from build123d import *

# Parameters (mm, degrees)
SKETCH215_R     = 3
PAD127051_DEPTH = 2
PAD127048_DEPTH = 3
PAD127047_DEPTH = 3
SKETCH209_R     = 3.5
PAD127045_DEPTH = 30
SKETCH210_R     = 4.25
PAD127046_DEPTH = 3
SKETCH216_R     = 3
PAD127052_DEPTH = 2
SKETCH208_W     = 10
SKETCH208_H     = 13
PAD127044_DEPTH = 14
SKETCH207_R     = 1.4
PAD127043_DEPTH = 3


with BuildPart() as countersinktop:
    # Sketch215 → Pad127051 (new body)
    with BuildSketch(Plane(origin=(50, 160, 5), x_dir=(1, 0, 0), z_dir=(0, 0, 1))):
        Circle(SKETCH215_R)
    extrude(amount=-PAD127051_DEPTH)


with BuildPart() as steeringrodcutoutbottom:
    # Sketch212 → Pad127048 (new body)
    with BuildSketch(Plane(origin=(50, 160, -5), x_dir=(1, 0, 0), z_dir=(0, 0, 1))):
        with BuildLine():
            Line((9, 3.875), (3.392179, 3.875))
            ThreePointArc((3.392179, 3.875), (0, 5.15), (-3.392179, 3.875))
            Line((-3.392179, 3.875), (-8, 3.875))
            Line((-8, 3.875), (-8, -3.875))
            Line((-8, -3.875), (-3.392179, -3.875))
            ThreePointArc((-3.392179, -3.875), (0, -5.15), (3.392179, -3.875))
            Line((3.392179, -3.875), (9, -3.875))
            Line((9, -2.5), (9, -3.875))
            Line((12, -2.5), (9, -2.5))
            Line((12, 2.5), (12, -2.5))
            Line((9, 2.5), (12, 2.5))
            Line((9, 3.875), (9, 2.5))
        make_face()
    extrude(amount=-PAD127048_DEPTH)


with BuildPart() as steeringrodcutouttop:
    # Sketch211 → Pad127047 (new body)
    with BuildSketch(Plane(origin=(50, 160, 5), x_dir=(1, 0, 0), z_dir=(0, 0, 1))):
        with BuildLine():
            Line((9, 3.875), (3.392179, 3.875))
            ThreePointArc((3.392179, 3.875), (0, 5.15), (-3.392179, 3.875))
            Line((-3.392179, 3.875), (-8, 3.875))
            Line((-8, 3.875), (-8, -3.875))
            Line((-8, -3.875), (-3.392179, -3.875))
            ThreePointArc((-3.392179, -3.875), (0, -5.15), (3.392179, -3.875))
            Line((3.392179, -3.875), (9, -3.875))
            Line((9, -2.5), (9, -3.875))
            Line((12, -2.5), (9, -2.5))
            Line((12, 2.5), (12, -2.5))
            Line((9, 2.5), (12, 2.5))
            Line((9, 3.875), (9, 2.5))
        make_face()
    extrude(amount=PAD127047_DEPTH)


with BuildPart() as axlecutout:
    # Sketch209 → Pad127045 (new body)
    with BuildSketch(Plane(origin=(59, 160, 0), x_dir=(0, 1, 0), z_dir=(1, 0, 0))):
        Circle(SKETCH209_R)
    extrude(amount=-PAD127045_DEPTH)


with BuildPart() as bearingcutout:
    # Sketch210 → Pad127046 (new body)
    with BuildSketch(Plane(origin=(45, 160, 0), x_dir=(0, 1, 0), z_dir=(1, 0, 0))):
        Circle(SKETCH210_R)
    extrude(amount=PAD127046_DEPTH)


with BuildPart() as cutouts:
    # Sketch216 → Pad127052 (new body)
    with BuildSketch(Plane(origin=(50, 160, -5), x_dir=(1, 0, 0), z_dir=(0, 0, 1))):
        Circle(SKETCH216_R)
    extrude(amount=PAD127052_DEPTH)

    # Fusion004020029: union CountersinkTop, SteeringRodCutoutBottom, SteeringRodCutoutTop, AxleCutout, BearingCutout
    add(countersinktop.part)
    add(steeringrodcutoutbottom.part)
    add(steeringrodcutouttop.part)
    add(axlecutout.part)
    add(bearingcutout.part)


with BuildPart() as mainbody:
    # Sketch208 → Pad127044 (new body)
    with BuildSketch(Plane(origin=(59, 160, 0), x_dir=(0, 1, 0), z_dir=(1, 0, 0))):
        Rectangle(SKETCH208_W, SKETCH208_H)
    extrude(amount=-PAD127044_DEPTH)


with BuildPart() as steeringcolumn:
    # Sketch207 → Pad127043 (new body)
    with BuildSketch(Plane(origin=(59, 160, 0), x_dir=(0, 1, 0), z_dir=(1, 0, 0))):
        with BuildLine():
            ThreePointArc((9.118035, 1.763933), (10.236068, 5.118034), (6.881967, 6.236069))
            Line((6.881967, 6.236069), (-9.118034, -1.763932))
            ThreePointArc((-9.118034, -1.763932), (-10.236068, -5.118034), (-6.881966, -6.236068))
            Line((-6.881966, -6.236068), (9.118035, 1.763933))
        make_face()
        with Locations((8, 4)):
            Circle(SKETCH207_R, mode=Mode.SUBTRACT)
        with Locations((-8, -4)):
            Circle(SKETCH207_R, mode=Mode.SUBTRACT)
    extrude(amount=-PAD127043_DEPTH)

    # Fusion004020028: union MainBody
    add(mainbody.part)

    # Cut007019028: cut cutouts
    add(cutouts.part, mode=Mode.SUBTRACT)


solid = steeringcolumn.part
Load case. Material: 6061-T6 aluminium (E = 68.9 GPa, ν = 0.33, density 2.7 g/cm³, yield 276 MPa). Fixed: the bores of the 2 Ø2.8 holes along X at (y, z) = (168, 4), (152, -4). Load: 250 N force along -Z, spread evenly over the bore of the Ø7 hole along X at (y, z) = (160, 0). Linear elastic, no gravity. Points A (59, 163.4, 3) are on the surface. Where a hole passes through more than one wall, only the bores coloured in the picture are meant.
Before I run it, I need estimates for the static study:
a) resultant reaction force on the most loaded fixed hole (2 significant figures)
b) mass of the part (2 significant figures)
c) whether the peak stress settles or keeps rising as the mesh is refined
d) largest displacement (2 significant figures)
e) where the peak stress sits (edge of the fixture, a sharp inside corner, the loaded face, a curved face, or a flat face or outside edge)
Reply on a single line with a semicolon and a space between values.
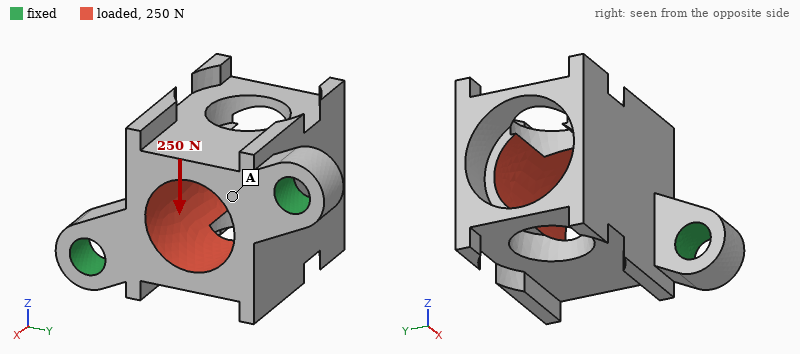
130 N; 2.4 g; keeps rising; 23 µm; edge of the fixture
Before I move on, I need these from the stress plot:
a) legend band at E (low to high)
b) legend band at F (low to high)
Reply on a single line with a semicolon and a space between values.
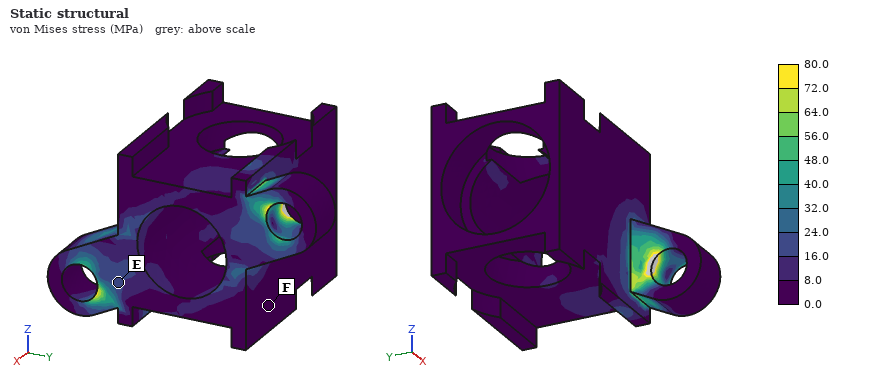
16.0 to 24.0 MPa; 0.0 to 8.0 MPa
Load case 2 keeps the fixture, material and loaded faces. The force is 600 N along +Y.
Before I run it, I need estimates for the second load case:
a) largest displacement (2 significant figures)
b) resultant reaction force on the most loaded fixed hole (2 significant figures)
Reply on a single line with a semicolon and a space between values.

35 µm; 330 N
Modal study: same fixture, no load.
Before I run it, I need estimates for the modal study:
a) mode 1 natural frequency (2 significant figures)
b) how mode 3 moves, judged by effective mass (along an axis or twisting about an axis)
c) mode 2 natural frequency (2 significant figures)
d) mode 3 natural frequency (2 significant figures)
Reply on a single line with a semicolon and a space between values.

10 kHz; along X; 25 kHz; 27 kHz
